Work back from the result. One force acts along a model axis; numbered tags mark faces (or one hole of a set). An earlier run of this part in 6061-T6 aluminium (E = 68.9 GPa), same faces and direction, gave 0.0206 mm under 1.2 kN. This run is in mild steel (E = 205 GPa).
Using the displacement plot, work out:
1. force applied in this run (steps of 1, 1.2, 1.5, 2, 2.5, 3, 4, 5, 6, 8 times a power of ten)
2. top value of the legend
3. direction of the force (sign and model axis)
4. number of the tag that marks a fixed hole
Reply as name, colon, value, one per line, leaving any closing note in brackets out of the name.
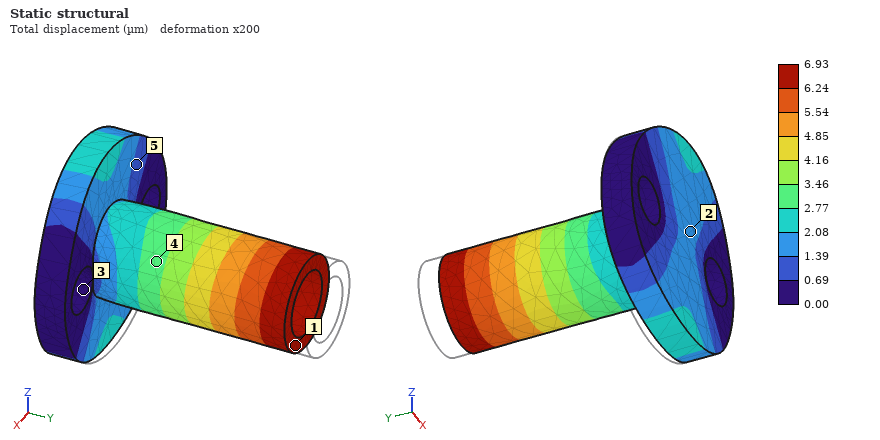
force applied in this run: 1.2 kN
top value of the legend: 6.93 µm
direction of the force: -Y
number of the tag that marks a fixed hole: 3
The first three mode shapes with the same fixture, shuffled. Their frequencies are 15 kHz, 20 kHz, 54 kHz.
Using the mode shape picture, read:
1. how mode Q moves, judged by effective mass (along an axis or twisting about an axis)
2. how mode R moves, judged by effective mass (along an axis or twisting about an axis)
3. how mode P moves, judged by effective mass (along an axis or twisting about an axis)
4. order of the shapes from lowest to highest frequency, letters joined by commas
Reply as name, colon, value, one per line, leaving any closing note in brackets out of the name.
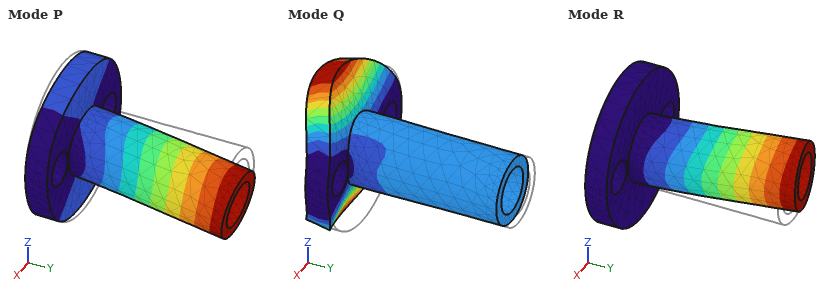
how mode Q moves, judged by effective mass: along Y
how mode R moves, judged by effective mass: along X
how mode P moves, judged by effective mass: along Z
order of the shapes from lowest to highest frequency, letters joined by commas: P, R, Q
